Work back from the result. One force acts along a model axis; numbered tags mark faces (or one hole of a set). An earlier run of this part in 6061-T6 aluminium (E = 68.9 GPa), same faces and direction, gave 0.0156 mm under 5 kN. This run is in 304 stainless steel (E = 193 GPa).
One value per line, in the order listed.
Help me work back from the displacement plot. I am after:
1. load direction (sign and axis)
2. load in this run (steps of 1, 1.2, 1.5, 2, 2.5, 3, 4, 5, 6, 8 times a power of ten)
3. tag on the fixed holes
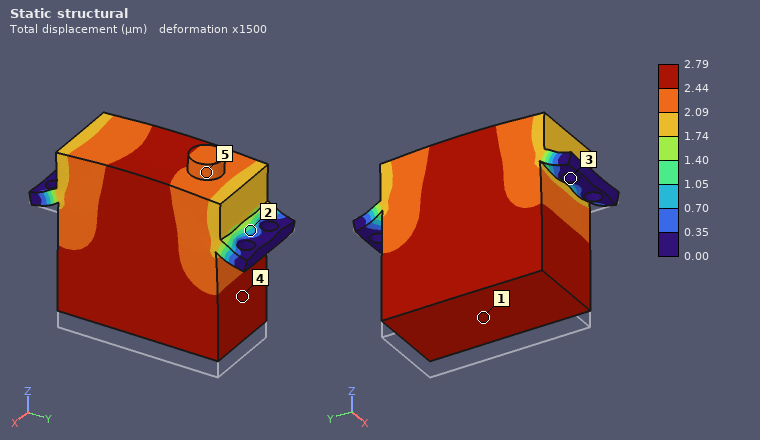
+Z
2.5 kN
3
